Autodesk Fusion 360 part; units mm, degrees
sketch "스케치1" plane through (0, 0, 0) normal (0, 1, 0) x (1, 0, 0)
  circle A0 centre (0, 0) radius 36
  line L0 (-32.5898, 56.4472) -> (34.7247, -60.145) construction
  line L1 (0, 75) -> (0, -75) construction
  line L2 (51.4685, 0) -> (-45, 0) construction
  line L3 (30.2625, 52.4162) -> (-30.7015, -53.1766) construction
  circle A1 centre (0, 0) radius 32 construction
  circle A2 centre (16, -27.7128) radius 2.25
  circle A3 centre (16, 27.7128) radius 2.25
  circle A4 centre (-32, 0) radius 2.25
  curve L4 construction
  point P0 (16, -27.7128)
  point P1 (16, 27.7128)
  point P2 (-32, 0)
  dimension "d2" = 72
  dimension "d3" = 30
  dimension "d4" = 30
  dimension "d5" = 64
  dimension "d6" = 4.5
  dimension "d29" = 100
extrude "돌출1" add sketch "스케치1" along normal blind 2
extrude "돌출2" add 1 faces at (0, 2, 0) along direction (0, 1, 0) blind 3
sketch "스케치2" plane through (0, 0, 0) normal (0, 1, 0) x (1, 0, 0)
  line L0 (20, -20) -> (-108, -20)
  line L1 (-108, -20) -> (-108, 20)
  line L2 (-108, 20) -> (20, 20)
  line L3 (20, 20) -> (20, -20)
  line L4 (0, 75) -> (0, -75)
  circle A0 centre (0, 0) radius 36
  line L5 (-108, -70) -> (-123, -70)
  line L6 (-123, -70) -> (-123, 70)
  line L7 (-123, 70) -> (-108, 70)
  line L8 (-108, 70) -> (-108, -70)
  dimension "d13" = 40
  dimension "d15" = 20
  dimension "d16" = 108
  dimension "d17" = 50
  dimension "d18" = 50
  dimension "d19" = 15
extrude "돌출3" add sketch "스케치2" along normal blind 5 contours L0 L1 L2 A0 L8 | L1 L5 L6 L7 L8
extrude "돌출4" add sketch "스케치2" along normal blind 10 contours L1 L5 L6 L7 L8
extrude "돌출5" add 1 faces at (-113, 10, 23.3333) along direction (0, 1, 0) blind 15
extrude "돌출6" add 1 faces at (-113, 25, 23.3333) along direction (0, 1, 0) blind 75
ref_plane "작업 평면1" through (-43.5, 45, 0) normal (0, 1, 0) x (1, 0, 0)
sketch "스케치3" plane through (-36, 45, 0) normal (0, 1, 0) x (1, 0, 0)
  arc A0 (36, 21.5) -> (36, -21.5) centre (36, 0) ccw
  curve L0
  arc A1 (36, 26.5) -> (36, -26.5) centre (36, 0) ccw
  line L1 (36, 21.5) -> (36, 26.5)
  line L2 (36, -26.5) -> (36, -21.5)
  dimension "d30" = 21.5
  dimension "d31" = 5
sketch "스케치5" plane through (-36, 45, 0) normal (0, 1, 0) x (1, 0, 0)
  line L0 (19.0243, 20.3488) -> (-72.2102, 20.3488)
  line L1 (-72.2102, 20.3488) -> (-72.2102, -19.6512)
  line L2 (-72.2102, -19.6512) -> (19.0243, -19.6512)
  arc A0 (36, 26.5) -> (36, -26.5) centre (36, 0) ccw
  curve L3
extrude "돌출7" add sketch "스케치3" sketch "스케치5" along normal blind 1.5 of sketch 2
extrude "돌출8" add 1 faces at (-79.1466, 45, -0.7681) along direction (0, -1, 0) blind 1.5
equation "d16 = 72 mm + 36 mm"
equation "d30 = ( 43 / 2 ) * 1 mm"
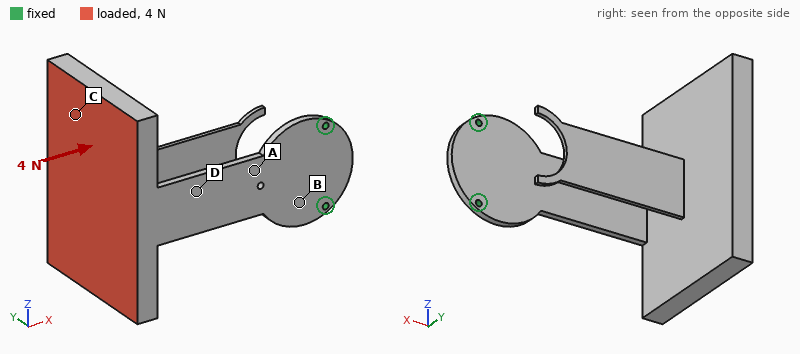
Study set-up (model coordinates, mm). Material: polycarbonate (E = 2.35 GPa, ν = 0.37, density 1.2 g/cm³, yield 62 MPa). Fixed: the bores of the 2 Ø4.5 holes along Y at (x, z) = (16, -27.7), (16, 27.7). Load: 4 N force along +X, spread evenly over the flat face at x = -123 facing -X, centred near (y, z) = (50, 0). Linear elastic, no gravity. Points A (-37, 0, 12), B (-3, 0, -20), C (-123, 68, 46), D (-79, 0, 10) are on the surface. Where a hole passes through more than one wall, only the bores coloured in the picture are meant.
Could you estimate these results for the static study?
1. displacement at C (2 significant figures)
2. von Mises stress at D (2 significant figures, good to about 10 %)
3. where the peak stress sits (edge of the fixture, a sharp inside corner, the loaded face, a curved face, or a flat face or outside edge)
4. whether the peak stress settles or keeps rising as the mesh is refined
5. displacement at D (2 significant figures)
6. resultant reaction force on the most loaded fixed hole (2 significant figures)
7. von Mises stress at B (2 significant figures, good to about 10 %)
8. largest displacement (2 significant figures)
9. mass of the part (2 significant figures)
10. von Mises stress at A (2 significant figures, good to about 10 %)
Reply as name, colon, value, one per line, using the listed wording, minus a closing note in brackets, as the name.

displacement at C: 2.1 mm
von Mises stress at D: 1.1 MPa
where the peak stress sits: edge of the fixture
whether the peak stress settles or keeps rising as the mesh is refined: keeps rising
displacement at D: 0.71 mm
resultant reaction force on the most loaded fixed hole: 2.0 N
von Mises stress at B: 0.61 MPa
largest displacement: 2.7 mm
mass of the part: 310 g
von Mises stress at A: 1.2 MPa
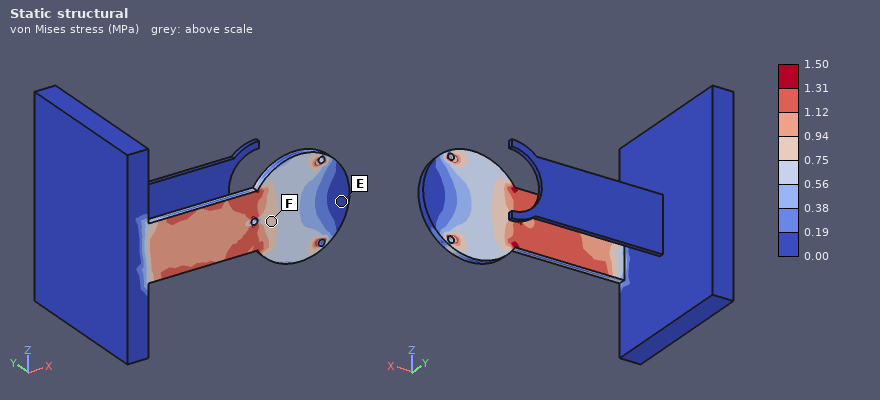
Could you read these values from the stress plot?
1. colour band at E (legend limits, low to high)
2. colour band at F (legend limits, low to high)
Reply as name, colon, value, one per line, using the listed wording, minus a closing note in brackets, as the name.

colour band at E: 0.00 to 0.19 MPa
colour band at F: 0.75 to 0.94 MPa
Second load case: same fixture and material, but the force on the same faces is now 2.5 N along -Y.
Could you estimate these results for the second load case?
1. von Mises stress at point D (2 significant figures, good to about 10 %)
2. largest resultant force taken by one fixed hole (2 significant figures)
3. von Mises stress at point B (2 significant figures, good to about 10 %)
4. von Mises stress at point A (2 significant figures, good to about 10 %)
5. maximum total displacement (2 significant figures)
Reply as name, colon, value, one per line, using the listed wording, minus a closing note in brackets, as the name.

von Mises stress at point D: 0.66 MPa
largest resultant force taken by one fixed hole: 1.3 N
von Mises stress at point B: 0.98 MPa
von Mises stress at point A: 1.4 MPa
maximum total displacement: 2.8 mm
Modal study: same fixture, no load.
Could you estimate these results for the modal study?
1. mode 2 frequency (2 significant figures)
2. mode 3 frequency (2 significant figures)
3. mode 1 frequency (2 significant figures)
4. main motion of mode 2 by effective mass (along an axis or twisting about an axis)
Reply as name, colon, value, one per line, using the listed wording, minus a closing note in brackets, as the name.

mode 2 frequency: 17 Hz
mode 3 frequency: 39 Hz
mode 1 frequency: 10 Hz
main motion of mode 2 by effective mass: along Z
